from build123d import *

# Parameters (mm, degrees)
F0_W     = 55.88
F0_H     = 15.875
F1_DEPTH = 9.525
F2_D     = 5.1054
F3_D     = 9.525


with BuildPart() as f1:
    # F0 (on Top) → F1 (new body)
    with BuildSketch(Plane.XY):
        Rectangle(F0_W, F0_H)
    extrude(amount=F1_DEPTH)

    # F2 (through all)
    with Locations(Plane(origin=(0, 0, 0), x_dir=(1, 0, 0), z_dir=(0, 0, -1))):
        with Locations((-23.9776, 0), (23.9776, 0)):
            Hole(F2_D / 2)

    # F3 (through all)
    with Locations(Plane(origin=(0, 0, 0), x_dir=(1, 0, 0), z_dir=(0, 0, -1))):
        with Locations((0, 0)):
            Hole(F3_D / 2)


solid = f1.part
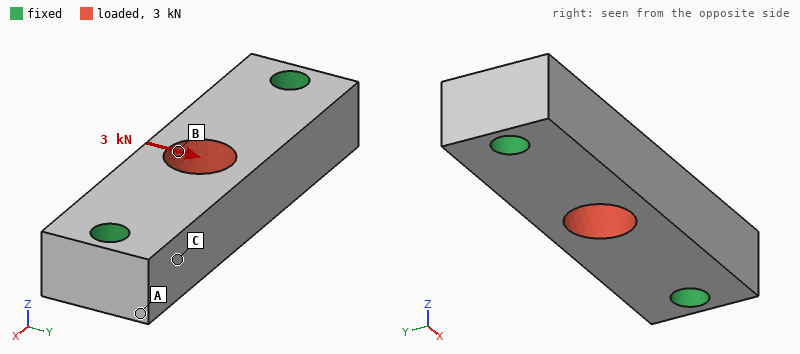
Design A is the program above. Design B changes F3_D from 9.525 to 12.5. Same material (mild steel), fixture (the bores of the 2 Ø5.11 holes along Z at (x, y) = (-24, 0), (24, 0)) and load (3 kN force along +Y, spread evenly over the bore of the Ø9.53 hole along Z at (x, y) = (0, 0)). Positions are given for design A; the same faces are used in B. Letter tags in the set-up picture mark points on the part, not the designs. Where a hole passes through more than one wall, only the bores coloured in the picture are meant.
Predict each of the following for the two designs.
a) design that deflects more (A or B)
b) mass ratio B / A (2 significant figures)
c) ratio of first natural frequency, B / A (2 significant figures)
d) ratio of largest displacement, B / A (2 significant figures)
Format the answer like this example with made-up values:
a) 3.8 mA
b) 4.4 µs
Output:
a) B
b) 0.93
c) 1.0
d) 1.1
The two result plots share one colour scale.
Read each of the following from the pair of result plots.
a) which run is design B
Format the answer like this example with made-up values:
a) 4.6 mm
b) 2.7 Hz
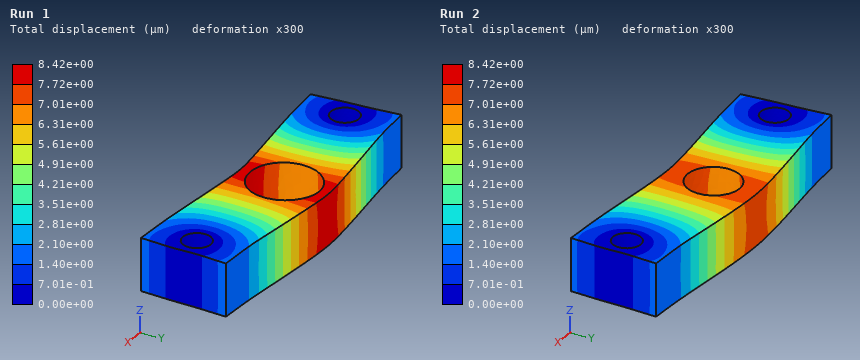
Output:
a) Run 1
